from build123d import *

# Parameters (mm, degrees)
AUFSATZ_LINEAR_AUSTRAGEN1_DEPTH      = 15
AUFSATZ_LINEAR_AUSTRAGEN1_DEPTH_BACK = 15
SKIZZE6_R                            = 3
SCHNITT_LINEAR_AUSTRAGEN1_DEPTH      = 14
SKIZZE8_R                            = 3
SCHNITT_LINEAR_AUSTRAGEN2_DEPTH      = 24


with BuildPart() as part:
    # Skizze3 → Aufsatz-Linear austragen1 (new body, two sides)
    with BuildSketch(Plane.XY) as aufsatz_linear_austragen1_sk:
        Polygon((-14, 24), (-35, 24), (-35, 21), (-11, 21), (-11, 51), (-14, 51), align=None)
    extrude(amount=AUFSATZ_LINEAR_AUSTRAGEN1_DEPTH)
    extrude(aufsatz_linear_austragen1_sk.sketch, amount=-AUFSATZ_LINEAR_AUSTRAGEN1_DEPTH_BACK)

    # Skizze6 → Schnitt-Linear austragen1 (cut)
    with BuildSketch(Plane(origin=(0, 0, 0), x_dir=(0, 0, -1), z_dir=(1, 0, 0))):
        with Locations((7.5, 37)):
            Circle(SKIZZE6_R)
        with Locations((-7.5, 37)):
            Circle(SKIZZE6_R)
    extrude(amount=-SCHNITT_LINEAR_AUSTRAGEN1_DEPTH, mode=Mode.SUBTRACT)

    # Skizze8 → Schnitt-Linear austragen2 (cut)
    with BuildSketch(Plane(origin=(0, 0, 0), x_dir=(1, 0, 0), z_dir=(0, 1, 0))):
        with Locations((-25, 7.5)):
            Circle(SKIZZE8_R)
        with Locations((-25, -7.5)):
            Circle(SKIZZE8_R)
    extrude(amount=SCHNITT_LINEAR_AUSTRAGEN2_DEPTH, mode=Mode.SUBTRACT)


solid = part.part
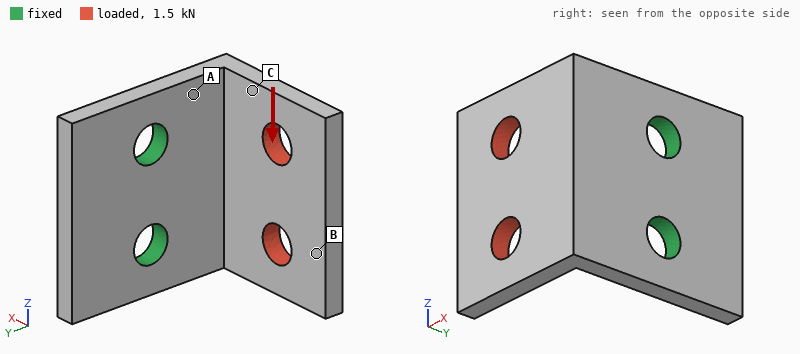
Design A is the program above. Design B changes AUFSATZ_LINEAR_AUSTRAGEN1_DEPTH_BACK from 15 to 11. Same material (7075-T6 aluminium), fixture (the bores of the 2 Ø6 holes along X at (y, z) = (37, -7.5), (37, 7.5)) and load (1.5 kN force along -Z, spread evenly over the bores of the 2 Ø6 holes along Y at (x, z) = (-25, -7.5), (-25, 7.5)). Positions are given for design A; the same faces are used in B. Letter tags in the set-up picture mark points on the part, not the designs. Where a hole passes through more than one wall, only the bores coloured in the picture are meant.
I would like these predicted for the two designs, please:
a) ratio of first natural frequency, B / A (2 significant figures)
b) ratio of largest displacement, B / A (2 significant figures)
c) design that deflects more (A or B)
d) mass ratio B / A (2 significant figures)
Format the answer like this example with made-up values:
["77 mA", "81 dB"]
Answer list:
["1.0", "1.2", "B", "0.86"]
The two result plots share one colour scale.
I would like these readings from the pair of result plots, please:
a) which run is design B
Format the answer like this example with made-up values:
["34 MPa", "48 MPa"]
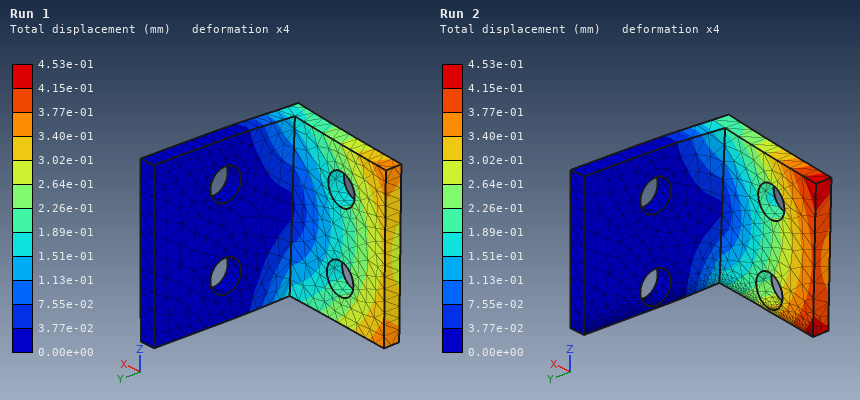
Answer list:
["Run 2"]
